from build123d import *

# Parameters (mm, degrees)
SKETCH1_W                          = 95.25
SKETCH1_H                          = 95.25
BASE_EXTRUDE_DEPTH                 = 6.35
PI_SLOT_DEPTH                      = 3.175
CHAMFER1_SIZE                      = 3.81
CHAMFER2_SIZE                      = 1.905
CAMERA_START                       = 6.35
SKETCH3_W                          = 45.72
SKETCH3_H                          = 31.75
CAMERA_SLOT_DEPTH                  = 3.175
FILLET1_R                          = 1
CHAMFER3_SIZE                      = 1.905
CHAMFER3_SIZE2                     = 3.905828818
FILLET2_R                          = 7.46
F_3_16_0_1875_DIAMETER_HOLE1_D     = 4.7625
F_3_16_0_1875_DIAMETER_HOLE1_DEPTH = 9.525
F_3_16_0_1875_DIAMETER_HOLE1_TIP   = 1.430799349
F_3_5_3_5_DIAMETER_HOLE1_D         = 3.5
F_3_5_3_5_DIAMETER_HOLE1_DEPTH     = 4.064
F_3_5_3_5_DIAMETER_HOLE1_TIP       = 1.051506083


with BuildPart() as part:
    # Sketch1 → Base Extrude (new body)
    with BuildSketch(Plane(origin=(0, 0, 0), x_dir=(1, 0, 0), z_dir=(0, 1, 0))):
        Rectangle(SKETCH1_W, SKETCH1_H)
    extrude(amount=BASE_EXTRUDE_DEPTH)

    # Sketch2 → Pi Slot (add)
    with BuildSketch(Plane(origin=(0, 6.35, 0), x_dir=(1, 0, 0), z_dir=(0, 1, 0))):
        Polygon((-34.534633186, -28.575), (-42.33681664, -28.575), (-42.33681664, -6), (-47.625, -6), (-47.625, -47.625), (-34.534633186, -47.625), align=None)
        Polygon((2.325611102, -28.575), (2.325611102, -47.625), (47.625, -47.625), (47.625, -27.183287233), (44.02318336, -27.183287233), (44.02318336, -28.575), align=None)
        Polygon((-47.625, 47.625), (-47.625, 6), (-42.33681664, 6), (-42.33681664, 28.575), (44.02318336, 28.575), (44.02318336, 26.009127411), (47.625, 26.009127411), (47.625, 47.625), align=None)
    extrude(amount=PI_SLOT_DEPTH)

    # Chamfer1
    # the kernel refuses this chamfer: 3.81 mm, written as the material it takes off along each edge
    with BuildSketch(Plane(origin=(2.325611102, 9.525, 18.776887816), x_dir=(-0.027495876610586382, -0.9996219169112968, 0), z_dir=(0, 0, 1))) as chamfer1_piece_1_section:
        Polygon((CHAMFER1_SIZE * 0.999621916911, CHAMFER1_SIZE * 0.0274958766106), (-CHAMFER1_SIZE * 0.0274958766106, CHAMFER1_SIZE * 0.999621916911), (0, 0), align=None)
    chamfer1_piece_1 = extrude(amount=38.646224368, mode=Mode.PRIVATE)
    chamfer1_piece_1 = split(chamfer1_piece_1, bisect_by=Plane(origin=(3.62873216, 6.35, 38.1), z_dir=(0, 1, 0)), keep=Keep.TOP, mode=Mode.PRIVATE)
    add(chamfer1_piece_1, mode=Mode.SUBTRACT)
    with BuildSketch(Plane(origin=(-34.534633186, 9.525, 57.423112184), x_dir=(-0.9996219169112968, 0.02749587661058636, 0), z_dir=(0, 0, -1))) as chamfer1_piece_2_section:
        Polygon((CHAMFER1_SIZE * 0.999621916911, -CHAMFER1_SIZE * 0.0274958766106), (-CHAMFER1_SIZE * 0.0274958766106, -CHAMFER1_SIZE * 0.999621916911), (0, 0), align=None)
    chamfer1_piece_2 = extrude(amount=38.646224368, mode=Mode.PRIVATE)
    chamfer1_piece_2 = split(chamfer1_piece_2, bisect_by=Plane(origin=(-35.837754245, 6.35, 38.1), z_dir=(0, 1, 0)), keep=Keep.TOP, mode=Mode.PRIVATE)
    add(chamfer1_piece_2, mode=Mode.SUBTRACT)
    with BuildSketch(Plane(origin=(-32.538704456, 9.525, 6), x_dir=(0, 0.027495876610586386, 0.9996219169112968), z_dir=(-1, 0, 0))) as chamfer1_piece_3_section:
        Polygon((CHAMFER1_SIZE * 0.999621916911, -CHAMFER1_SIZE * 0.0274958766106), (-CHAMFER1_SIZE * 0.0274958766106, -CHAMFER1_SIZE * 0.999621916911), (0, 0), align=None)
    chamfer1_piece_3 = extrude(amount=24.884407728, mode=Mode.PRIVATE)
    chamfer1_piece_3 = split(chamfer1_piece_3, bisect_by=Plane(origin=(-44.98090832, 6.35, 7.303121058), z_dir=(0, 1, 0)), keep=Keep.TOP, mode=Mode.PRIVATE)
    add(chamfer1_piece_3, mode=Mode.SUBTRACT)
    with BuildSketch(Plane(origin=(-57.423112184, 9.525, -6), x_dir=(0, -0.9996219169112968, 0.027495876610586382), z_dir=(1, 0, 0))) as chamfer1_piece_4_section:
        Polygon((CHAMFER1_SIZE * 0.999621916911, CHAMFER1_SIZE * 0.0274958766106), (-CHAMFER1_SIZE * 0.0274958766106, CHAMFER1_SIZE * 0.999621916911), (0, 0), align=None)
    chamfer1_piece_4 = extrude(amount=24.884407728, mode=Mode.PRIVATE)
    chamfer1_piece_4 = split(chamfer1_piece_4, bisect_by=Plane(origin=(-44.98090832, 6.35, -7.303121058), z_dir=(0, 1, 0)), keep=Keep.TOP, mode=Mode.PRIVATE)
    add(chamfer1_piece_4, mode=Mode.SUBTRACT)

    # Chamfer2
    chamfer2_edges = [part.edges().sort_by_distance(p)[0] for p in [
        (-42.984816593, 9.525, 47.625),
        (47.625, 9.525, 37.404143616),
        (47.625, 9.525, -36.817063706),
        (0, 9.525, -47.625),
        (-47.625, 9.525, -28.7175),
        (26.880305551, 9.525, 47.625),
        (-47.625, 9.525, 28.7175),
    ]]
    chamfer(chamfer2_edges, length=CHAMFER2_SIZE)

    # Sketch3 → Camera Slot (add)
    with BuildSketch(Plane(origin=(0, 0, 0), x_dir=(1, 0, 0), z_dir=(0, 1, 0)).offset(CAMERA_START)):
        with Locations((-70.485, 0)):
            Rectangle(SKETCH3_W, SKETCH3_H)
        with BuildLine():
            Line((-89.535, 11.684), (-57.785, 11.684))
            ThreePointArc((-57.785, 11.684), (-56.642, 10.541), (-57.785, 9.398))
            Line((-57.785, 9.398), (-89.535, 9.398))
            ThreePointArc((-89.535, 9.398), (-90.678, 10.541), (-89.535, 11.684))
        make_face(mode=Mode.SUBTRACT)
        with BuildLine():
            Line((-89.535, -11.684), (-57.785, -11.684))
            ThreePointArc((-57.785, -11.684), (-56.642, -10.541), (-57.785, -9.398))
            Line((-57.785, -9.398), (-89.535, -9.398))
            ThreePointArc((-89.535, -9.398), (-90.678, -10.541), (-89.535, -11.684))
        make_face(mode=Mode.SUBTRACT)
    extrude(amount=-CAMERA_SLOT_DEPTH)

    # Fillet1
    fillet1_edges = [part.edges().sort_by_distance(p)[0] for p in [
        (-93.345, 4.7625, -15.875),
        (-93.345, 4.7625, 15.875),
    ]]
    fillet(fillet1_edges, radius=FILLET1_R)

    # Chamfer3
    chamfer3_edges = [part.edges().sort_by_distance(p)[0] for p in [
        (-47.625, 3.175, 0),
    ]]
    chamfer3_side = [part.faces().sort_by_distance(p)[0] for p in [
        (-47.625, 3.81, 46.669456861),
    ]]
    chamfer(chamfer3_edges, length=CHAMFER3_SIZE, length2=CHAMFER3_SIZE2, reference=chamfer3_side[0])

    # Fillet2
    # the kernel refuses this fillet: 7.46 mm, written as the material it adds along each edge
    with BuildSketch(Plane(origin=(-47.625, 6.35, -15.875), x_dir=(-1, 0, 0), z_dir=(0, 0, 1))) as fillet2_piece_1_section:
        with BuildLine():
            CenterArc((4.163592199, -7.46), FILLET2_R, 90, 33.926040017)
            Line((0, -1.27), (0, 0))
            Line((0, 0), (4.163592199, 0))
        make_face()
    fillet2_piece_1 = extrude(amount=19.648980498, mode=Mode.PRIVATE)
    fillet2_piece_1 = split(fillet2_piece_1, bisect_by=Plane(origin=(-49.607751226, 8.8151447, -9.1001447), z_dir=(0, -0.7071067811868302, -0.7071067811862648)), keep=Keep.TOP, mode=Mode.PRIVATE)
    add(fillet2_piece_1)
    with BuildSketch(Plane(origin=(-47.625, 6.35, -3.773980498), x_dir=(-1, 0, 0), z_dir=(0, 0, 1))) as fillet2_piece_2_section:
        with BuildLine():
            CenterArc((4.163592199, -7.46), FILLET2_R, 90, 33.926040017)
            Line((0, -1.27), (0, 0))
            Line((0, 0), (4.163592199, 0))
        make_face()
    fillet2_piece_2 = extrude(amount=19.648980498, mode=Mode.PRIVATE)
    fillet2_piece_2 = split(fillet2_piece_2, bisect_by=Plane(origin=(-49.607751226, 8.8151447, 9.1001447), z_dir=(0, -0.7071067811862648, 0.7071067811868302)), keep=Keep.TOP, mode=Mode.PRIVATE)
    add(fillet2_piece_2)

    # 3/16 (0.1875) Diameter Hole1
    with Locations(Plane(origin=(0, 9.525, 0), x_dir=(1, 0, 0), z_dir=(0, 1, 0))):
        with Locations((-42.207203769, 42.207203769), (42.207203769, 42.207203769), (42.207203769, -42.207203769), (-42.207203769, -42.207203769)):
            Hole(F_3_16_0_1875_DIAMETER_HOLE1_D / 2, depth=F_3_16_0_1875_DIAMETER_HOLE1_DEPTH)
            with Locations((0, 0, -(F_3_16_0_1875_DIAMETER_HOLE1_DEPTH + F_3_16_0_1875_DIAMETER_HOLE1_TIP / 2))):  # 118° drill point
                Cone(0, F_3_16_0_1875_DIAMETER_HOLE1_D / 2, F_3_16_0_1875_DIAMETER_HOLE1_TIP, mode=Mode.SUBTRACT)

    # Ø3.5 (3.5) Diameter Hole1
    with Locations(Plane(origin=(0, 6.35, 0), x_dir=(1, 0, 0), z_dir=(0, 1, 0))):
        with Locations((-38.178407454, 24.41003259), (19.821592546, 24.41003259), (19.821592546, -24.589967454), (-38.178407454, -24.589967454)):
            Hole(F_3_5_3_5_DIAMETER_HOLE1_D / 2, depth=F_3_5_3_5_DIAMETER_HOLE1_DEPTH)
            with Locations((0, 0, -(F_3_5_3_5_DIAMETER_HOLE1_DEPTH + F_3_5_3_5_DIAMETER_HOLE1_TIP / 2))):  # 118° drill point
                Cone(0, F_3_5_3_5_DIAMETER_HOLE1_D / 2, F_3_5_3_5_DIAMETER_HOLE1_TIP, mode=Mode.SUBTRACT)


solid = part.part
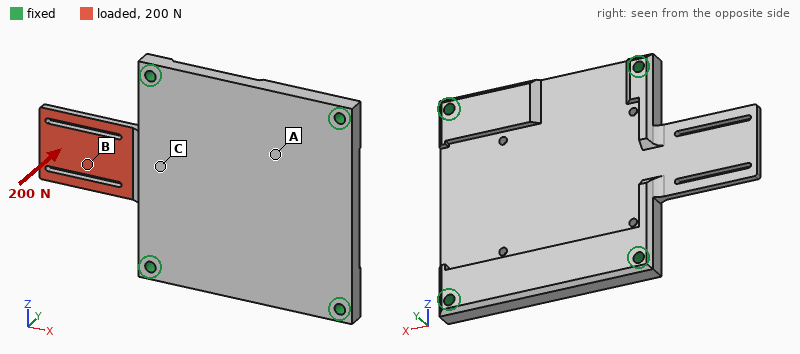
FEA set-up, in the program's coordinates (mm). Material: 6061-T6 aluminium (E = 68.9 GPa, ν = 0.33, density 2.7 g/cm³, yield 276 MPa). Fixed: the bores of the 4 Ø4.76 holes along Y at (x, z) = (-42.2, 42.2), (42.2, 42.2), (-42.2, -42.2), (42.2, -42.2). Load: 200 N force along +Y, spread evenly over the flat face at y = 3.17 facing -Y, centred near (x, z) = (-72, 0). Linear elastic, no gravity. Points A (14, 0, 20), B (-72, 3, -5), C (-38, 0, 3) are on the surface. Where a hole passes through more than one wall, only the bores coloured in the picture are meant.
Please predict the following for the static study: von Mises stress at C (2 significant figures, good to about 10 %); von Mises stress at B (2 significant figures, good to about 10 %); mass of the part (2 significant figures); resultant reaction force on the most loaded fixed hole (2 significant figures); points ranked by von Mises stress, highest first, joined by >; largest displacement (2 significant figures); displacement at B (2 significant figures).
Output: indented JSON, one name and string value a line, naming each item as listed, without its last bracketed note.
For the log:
{
  "von Mises stress at C": "15 MPa",
  "von Mises stress at B": "25 MPa",
  "mass of the part": "190 g",
  "resultant reaction force on the most loaded fixed hole": "180 N",
  "points ranked by von Mises stress, highest first, joined by >": "B > C > A",
  "largest displacement": "0.51 mm",
  "displacement at B": "0.21 mm"
}
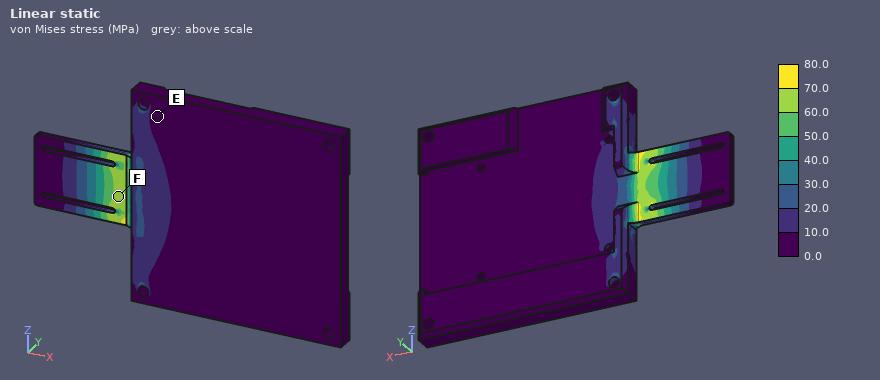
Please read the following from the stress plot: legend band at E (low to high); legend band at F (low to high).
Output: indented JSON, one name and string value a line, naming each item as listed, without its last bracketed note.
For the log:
{
  "legend band at E": "0.0 to 10.0 MPa",
  "legend band at F": "60.0 to 70.0 MPa"
}
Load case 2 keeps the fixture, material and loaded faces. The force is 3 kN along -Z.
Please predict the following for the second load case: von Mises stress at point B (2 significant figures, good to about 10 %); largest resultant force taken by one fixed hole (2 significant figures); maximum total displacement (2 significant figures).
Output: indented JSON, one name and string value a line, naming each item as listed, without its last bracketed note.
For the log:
{
  "von Mises stress at point B": "100 MPa",
  "largest resultant force taken by one fixed hole": "1.6 kN",
  "maximum total displacement": "0.35 mm"
}
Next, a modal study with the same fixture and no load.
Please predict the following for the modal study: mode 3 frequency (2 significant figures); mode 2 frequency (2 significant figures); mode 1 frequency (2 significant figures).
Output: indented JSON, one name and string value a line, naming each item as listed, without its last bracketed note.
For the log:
{
  "mode 3 frequency": "3800 Hz",
  "mode 2 frequency": "3600 Hz",
  "mode 1 frequency": "1200 Hz"
}
